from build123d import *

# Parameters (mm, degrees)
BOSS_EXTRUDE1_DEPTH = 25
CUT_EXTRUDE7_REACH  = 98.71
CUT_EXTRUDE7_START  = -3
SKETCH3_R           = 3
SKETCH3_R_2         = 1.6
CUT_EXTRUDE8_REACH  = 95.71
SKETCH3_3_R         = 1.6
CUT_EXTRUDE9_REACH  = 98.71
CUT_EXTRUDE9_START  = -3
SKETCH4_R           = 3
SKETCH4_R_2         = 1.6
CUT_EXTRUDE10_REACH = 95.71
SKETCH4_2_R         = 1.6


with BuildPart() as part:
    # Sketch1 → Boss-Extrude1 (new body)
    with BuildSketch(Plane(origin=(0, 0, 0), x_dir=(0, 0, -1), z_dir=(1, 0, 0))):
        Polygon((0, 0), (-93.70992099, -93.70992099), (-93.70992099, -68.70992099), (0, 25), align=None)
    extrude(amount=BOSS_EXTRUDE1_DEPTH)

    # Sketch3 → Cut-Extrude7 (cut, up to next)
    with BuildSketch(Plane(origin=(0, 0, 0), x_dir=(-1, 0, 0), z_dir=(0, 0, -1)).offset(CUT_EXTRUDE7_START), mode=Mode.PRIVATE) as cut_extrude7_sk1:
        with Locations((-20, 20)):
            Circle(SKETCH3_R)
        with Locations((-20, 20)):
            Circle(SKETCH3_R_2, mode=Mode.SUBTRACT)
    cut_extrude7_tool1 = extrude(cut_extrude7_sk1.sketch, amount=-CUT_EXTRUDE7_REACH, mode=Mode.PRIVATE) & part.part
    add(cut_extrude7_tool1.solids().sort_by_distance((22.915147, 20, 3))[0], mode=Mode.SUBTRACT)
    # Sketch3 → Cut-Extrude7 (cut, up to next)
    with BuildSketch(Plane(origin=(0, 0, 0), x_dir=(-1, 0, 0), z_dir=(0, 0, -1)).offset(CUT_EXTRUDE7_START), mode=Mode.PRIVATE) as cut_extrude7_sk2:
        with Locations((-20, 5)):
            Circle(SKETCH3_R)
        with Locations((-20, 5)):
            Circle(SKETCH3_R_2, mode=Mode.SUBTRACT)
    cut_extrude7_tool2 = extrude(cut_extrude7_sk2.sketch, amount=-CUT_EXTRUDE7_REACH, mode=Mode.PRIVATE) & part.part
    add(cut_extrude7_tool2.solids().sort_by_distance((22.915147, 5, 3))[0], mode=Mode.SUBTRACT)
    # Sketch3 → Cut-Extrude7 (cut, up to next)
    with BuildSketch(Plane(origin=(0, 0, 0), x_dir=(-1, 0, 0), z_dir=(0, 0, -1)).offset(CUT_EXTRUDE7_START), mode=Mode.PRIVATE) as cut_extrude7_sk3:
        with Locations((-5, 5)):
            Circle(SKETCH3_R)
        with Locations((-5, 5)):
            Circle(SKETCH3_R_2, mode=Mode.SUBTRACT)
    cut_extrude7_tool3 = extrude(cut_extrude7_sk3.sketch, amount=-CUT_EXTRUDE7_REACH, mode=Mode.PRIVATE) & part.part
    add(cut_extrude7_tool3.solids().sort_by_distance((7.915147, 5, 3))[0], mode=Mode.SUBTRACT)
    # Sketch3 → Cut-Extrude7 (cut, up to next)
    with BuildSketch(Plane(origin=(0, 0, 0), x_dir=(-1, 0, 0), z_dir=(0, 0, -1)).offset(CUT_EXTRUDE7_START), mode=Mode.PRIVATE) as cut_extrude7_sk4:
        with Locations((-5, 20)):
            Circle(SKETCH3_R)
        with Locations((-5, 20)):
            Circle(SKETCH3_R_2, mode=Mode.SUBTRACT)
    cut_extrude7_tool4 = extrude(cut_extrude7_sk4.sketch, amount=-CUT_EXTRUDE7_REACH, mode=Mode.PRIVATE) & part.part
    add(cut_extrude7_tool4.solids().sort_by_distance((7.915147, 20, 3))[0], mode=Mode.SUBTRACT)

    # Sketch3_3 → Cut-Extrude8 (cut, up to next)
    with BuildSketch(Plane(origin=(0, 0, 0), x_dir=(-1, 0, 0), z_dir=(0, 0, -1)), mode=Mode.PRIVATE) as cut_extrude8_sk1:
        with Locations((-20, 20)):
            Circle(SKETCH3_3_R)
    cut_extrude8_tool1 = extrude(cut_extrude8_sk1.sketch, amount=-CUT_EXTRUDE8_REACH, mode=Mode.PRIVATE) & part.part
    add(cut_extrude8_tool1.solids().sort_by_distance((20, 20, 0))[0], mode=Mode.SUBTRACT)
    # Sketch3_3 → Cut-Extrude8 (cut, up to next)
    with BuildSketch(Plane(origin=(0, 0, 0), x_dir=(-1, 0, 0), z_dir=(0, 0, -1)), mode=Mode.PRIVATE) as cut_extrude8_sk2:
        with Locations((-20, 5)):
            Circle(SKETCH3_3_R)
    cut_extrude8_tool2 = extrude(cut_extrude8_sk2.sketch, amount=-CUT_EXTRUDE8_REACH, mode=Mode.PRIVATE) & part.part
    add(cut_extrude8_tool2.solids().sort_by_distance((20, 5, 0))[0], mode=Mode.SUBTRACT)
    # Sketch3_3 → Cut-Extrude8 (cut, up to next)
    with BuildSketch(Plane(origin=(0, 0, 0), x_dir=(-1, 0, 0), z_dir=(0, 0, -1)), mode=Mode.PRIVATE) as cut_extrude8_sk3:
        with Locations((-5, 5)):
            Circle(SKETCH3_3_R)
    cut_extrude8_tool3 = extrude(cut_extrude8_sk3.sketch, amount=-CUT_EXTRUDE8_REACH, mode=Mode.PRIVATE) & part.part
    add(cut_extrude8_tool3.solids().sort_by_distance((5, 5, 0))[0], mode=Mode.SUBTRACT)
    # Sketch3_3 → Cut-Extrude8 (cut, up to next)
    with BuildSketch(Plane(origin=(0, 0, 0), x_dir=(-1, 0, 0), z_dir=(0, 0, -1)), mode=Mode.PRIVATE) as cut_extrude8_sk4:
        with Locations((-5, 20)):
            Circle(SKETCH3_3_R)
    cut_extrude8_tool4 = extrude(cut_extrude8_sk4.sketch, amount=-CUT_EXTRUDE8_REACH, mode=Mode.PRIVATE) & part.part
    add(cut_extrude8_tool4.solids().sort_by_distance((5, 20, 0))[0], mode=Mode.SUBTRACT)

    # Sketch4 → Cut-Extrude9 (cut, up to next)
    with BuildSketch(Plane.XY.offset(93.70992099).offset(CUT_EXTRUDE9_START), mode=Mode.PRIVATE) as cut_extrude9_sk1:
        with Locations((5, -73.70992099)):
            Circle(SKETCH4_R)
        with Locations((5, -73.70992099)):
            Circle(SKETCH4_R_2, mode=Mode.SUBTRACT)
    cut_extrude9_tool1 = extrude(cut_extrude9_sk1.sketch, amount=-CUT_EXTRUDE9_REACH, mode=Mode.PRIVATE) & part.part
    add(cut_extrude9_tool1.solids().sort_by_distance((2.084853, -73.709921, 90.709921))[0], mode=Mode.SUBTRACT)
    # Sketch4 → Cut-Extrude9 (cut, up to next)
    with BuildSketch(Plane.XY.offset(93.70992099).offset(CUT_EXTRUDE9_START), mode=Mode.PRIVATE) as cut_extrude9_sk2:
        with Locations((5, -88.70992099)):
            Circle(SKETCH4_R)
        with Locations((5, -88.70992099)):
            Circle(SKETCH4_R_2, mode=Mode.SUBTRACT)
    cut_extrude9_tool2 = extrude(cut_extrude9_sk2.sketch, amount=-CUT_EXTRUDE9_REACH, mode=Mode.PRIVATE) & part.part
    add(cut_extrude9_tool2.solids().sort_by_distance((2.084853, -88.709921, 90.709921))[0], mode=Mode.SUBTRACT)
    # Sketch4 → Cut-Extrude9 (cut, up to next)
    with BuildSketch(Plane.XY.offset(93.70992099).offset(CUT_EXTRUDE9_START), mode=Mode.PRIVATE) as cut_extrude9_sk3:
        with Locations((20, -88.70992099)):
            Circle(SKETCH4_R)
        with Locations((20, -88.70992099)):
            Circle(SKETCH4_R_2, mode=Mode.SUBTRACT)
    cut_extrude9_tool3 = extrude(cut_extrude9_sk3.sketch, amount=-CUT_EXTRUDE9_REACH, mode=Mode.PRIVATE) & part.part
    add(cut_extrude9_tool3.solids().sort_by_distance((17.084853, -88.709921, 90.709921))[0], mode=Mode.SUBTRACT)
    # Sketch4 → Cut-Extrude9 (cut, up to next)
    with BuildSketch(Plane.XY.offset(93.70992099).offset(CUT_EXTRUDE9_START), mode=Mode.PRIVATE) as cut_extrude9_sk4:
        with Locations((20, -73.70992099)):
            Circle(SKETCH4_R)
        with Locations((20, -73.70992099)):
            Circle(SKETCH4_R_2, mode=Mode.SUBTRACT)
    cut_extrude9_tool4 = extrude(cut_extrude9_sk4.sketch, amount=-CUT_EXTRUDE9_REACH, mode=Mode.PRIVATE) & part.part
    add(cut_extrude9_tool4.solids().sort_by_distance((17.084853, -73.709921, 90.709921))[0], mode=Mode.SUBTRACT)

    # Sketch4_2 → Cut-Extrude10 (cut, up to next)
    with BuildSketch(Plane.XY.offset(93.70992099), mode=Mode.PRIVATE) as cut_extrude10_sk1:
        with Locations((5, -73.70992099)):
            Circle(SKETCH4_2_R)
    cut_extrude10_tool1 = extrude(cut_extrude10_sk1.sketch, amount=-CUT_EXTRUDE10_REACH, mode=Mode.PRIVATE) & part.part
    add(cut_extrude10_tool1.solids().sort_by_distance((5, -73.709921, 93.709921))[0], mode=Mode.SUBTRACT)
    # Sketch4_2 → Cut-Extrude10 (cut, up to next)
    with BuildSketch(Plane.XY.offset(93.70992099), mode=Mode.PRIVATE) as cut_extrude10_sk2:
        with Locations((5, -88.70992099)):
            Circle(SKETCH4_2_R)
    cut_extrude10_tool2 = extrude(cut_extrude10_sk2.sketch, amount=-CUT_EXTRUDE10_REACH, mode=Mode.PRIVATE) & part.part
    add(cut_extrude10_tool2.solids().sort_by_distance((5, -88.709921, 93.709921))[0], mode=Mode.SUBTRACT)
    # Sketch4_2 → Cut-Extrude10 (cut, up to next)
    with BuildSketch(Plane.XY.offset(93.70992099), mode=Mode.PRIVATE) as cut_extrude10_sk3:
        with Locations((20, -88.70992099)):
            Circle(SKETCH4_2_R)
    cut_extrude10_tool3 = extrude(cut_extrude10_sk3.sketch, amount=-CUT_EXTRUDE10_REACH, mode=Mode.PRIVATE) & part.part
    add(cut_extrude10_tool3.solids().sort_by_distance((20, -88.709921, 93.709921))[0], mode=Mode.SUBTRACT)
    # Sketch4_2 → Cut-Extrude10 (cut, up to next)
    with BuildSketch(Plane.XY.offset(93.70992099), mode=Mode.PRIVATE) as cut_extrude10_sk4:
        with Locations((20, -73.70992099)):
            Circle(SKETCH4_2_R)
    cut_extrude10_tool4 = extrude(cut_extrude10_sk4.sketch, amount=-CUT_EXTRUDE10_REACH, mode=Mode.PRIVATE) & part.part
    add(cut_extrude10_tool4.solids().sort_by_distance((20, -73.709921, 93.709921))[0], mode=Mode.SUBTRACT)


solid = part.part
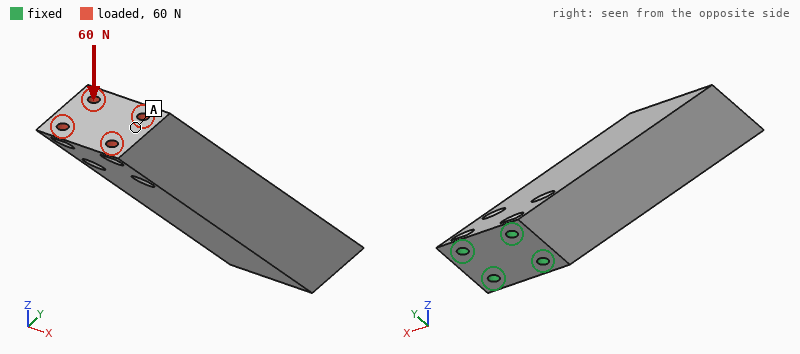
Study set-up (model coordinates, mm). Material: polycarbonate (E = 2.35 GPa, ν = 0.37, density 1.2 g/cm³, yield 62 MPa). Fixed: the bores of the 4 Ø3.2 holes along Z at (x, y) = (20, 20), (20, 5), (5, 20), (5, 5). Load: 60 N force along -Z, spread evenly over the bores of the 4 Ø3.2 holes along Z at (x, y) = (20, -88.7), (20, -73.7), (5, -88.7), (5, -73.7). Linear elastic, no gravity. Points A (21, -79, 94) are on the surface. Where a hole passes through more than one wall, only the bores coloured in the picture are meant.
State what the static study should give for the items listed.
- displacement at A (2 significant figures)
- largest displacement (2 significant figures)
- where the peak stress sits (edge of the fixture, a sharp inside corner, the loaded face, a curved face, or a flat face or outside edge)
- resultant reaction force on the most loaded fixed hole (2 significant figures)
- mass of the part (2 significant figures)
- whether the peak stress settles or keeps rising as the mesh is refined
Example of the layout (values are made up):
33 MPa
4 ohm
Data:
1.6 mm
1.8 mm
edge of the fixture
210 N
67 g
keeps rising
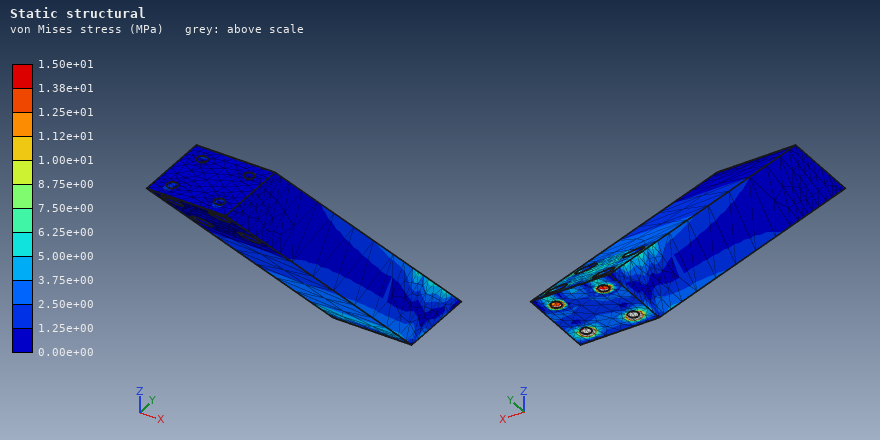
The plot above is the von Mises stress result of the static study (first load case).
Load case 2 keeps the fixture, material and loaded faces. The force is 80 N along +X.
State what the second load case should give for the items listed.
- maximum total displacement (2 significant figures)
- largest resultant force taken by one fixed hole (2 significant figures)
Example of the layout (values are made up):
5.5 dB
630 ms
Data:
1.7 mm
400 N
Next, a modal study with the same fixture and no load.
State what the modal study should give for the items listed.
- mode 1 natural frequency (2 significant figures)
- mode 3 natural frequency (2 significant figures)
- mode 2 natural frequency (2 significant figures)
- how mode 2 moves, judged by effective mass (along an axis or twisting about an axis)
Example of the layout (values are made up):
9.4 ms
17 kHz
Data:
190 Hz
1200 Hz
270 Hz
along X
